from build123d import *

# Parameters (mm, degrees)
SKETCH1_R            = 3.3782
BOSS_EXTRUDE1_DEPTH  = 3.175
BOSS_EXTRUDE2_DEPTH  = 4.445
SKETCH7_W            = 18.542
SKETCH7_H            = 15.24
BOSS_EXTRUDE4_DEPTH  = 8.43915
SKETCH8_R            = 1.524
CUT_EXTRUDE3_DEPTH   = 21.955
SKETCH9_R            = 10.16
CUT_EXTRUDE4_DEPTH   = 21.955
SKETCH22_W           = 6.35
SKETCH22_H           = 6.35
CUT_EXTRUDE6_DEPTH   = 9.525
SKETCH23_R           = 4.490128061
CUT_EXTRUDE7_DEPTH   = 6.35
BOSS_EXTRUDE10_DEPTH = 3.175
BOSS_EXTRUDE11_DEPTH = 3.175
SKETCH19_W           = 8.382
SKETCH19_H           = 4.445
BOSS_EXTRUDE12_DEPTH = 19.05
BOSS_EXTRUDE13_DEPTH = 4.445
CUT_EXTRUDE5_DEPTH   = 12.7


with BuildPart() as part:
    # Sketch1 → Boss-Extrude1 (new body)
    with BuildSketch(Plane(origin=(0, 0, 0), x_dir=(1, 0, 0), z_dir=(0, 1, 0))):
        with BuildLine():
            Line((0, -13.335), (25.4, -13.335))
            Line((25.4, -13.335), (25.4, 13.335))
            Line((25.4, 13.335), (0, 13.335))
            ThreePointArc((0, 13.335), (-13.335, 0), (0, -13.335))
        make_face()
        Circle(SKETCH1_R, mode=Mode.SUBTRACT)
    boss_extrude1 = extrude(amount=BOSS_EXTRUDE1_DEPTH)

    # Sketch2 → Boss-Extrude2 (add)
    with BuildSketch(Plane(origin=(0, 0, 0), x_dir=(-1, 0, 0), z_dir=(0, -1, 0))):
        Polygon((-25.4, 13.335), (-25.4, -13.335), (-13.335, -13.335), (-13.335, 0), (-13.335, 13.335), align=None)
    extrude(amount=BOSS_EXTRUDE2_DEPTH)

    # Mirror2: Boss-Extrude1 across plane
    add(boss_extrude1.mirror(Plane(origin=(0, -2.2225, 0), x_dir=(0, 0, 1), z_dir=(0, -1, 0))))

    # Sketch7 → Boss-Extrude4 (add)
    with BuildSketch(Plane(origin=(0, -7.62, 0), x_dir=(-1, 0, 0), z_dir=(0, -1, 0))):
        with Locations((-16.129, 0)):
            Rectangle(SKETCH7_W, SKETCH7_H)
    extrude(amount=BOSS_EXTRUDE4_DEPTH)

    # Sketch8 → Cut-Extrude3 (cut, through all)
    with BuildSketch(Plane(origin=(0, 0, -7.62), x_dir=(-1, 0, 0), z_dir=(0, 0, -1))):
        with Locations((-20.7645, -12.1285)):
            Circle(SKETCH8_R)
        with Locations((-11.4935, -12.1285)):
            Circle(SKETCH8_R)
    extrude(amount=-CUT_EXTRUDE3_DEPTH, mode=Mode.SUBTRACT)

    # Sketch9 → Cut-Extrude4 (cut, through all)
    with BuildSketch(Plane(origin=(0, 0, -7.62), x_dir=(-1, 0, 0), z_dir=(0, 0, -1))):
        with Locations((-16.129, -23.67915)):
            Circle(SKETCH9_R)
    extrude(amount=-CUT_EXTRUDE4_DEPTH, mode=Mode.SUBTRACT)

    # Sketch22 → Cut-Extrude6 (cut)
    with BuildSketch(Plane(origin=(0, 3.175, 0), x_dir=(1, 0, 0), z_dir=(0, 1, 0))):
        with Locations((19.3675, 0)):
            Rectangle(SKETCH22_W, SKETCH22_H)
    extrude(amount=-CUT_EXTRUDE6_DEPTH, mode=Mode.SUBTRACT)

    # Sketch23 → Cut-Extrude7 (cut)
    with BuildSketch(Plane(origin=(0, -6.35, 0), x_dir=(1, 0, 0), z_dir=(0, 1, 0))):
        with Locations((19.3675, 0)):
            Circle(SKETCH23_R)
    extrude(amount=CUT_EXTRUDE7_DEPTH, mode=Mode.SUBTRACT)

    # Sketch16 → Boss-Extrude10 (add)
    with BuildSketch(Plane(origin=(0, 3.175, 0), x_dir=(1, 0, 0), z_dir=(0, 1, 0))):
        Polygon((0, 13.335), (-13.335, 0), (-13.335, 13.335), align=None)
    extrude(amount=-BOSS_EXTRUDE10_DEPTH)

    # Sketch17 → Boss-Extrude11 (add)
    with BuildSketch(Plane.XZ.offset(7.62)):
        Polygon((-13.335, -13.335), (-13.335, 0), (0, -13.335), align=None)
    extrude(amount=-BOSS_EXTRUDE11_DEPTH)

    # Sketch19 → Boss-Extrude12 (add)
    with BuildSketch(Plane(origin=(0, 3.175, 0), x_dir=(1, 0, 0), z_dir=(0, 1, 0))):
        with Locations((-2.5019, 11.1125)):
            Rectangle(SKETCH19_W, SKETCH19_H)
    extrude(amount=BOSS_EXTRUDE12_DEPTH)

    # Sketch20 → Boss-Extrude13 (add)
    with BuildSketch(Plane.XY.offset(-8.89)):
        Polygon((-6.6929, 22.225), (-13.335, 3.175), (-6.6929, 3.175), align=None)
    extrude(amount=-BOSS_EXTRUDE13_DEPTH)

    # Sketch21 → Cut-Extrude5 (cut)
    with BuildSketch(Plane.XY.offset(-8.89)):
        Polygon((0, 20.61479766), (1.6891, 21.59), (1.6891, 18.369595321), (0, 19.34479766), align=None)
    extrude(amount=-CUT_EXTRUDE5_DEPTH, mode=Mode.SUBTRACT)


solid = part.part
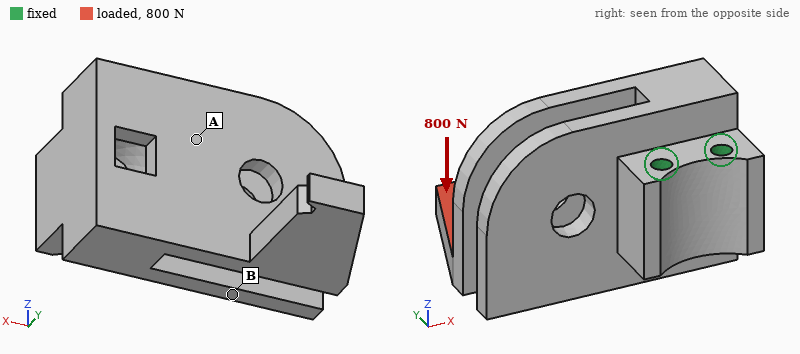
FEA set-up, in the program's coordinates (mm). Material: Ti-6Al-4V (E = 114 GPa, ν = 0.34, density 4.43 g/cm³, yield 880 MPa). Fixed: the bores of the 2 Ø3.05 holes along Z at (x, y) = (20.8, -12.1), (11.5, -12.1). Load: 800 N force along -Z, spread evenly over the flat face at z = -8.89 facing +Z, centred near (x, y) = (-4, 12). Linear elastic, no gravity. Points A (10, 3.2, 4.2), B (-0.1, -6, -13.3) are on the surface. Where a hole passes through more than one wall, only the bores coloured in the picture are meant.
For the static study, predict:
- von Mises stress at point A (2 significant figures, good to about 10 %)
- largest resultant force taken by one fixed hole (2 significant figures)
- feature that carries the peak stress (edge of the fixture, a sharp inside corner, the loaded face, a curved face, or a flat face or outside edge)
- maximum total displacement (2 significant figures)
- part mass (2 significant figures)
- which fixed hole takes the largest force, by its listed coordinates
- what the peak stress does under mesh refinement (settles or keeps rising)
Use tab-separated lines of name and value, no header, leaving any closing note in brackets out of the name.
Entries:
von Mises stress at point A	66 MPa
largest resultant force taken by one fixed hole	1.2 kN
feature that carries the peak stress	a sharp inside corner
maximum total displacement	0.42 mm
part mass	43 g
which fixed hole takes the largest force, by its listed coordinates	(11.5, -12.1)
what the peak stress does under mesh refinement	keeps rising
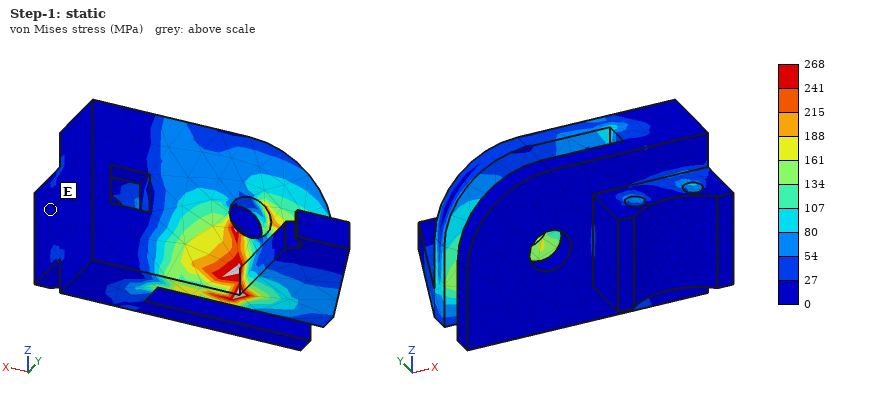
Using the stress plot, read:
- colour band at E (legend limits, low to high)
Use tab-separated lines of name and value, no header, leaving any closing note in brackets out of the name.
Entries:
colour band at E	0 to 27 MPa
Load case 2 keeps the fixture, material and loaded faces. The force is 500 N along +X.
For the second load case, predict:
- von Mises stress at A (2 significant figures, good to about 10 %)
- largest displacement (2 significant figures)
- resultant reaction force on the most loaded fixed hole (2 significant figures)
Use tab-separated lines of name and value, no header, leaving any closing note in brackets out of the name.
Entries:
von Mises stress at A	94 MPa
largest displacement	0.36 mm
resultant reaction force on the most loaded fixed hole	1.1 kN
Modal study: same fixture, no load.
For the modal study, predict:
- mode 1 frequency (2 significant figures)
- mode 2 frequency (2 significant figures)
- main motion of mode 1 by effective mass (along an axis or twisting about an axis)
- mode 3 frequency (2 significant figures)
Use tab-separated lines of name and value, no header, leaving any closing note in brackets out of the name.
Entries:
mode 1 frequency	2100 Hz
mode 2 frequency	4000 Hz
main motion of mode 1 by effective mass	along Y
mode 3 frequency	5300 Hz
